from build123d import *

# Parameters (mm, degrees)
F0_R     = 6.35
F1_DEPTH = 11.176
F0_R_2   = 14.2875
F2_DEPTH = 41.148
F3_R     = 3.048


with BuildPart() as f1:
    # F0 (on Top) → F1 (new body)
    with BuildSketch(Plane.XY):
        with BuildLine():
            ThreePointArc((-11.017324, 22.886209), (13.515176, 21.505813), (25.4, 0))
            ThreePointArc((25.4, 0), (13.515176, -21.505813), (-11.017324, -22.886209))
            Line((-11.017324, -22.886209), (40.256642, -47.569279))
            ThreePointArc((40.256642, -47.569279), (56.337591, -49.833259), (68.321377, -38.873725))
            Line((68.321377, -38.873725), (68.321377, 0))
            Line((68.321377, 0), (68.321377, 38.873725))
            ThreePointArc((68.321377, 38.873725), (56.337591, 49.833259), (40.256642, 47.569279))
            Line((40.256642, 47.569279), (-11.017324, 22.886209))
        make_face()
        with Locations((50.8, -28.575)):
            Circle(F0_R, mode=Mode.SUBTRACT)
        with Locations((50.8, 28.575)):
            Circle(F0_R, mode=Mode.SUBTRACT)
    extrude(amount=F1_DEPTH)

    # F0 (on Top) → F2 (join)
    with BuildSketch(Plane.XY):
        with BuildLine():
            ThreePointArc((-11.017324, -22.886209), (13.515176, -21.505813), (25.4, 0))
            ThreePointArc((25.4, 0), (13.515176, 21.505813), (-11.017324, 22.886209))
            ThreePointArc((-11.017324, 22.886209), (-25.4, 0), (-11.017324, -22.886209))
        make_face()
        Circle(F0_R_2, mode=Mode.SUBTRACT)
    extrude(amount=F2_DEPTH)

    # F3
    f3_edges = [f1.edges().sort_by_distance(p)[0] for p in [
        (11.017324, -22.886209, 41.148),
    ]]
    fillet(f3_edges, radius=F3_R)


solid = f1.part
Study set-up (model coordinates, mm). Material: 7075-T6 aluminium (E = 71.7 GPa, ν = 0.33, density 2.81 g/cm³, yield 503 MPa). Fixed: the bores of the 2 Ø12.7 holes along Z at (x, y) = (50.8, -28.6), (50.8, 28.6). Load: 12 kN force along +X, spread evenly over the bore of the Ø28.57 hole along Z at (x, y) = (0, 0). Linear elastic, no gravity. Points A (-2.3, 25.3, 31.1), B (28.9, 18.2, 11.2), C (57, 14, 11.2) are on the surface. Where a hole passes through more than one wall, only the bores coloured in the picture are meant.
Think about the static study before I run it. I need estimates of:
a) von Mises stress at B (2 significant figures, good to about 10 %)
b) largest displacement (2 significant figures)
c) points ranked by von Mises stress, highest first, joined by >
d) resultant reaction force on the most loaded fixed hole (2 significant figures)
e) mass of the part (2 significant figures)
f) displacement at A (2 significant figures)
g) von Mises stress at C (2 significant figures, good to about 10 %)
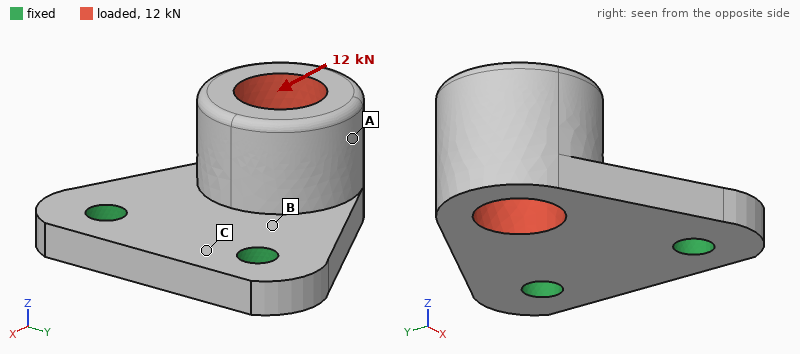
110 MPa
0.59 mm
B > C > A
6.3 kN
300 g
0.38 mm
26 MPa
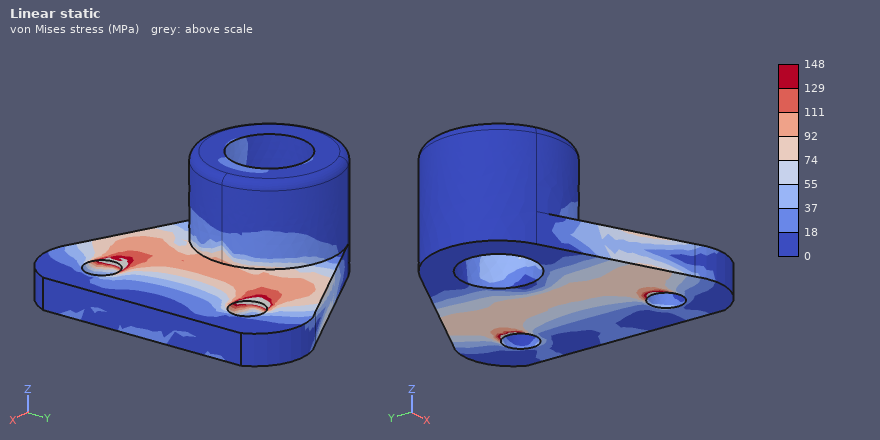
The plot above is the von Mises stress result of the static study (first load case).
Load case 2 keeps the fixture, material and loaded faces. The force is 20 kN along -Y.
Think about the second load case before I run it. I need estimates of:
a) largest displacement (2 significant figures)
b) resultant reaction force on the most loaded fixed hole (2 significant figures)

0.25 mm
19 kN
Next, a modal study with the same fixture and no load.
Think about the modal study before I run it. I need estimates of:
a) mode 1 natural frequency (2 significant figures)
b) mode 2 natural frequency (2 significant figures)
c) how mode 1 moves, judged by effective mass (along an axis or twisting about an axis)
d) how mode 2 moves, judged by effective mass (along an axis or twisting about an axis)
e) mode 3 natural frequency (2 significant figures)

1400 Hz
3800 Hz
along Z
along Y
6400 Hz
